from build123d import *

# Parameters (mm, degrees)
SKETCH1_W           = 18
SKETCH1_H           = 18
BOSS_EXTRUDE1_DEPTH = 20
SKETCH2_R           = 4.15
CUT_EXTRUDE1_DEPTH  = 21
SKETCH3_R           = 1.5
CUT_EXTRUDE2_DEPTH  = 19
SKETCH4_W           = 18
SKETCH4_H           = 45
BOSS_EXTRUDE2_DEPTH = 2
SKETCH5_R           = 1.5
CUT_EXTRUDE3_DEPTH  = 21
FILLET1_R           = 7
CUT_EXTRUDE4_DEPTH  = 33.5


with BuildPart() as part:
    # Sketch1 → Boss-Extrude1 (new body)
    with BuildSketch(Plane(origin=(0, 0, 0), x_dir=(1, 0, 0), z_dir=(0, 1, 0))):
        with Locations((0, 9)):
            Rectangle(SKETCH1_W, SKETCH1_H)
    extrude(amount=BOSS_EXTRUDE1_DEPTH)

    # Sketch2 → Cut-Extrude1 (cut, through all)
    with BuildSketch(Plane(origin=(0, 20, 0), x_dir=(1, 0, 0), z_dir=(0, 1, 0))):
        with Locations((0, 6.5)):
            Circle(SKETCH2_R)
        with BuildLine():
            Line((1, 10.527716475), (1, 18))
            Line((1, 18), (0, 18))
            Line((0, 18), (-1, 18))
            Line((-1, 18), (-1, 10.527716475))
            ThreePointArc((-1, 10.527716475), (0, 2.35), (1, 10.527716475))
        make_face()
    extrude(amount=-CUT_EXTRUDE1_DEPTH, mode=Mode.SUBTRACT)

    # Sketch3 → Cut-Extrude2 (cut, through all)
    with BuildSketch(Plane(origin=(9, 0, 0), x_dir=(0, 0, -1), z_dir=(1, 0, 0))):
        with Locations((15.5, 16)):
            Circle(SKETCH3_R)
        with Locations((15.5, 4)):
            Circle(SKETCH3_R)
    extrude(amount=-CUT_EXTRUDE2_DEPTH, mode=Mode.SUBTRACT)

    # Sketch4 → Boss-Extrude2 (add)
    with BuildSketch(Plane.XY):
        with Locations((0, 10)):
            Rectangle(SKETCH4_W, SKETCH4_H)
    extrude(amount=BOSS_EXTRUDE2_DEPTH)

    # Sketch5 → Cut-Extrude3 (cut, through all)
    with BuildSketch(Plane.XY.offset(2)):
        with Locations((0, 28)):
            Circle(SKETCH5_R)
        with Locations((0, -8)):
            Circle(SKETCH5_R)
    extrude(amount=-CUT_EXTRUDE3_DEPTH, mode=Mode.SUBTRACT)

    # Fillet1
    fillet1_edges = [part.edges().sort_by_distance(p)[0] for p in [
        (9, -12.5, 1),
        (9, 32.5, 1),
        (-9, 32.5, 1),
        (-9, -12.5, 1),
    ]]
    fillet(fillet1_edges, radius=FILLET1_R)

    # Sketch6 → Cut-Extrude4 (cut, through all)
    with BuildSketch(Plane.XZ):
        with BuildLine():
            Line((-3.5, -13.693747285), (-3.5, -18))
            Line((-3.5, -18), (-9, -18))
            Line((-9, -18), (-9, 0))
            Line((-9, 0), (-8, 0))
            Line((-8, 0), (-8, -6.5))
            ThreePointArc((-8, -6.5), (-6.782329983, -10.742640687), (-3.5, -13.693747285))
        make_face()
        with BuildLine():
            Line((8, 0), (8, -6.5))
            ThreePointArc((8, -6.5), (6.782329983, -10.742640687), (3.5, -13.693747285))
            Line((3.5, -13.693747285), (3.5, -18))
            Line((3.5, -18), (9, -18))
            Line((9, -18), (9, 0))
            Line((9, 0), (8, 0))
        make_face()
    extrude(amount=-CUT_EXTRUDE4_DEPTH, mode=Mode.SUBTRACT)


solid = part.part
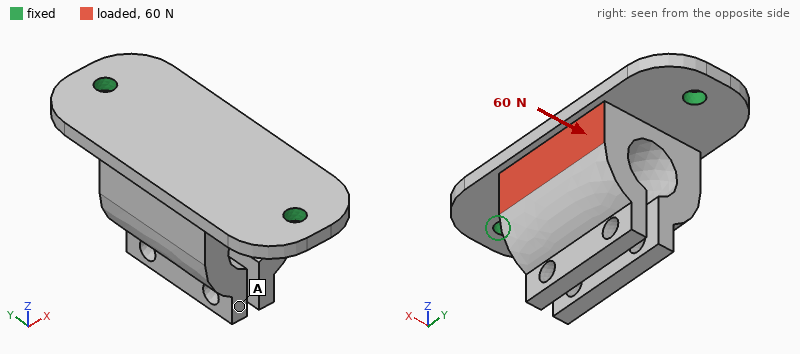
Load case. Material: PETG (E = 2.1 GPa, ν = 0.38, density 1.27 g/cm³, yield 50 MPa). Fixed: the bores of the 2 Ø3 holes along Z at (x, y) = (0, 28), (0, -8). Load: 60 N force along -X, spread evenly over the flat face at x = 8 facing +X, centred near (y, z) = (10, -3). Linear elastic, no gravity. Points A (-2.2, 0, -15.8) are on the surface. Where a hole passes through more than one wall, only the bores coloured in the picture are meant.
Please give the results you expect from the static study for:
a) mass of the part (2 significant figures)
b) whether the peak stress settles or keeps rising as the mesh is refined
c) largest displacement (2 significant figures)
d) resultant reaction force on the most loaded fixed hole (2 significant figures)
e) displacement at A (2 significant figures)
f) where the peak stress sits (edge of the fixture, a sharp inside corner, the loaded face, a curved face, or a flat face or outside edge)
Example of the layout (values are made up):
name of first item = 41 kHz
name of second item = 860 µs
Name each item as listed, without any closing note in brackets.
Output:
mass of the part = 5.9 g
whether the peak stress settles or keeps rising as the mesh is refined = keeps rising
largest displacement = 0.48 mm
resultant reaction force on the most loaded fixed hole = 30 N
displacement at A = 0.39 mm
where the peak stress sits = edge of the fixture
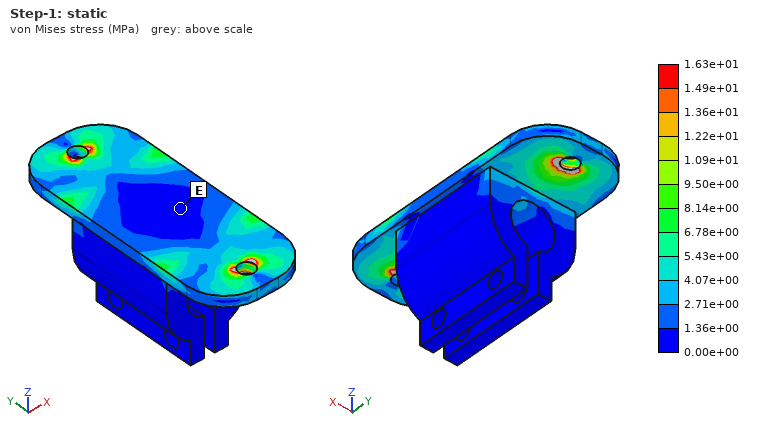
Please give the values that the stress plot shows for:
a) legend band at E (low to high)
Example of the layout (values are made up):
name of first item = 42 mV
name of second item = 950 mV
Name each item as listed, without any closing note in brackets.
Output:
legend band at E = 0.00e+00 to 1.36e+00 MPa
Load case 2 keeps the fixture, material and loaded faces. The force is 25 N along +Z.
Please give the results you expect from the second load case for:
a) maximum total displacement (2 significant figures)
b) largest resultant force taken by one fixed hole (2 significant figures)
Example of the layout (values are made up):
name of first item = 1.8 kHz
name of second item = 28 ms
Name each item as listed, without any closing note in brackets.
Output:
maximum total displacement = 0.36 mm
largest resultant force taken by one fixed hole = 15 N
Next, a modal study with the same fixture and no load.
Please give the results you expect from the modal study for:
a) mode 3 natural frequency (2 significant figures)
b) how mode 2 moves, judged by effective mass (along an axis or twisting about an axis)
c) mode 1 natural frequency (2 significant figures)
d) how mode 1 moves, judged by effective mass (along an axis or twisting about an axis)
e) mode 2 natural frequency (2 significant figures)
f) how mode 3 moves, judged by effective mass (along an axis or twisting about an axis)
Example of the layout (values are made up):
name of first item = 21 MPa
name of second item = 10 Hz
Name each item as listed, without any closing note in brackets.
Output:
mode 3 natural frequency = 2200 Hz
how mode 2 moves, judged by effective mass = along Z
mode 1 natural frequency = 750 Hz
how mode 1 moves, judged by effective mass = along X
mode 2 natural frequency = 1700 Hz
how mode 3 moves, judged by effective mass = along Y
